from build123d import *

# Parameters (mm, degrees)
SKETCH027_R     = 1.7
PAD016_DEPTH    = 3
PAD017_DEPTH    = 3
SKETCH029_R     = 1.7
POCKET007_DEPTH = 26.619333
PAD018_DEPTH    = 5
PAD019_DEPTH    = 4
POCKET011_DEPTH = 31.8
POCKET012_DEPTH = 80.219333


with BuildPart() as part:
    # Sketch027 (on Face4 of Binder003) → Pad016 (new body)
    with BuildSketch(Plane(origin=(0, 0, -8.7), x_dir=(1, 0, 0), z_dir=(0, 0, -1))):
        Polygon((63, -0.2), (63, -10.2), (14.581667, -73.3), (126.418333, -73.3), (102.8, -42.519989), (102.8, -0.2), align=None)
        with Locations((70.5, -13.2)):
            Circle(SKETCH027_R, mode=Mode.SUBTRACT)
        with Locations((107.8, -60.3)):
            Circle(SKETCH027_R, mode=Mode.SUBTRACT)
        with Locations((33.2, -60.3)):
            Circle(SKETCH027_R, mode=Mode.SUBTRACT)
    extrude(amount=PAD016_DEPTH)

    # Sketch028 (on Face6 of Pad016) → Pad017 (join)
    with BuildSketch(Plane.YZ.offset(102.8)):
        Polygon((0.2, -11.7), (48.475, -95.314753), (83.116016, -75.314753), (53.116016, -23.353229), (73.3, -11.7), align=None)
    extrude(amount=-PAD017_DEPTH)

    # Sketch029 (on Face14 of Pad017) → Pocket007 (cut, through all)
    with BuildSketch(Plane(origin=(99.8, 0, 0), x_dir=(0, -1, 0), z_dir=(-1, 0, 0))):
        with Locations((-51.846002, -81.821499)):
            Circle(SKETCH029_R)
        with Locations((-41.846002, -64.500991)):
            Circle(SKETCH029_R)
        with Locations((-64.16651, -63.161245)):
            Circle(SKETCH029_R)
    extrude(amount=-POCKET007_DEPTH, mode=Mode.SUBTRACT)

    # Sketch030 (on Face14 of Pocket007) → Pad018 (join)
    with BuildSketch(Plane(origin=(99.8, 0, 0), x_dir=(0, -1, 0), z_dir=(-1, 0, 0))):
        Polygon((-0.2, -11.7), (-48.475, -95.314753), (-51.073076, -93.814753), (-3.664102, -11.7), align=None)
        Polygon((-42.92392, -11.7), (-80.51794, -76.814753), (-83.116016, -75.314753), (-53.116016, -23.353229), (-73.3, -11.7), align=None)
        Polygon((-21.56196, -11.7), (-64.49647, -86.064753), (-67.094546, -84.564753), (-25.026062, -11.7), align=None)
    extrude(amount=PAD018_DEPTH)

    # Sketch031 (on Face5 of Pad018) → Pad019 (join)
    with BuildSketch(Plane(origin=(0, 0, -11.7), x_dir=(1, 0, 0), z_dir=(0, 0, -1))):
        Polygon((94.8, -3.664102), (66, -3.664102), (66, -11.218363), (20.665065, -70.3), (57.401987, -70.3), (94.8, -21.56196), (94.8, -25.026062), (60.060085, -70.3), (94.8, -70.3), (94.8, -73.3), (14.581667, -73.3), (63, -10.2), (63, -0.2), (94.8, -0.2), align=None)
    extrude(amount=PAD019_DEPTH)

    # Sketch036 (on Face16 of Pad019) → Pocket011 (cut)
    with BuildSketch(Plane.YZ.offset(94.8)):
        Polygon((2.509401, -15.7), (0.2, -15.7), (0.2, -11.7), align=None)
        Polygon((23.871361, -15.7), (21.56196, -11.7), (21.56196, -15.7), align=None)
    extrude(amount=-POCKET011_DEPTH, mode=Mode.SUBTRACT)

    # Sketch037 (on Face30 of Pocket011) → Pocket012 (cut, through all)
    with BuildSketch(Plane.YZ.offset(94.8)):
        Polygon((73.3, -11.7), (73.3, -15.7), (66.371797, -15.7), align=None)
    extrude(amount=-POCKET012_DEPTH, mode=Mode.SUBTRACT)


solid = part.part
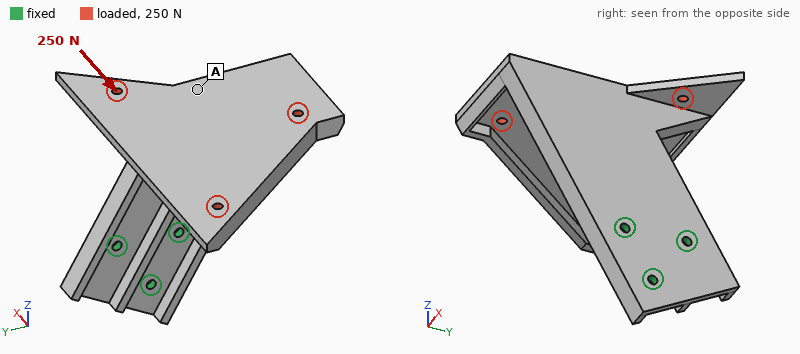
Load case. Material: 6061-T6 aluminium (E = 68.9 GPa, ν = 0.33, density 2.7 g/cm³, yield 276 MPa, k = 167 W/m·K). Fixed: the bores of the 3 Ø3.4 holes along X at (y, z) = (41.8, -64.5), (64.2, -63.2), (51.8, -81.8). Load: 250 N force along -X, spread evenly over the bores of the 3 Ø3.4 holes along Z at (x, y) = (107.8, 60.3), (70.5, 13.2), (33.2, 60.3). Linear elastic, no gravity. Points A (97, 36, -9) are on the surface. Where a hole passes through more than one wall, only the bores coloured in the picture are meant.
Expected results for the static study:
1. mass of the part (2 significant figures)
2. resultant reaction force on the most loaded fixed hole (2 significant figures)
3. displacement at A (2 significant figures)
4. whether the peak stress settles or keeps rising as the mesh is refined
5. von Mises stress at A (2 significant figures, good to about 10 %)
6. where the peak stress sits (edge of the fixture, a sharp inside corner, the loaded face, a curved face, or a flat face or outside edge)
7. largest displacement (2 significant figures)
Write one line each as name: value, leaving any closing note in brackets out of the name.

mass of the part: 85 g
resultant reaction force on the most loaded fixed hole: 400 N
displacement at A: 0.60 mm
whether the peak stress settles or keeps rising as the mesh is refined: keeps rising
von Mises stress at A: 13 MPa
where the peak stress sits: edge of the fixture
largest displacement: 1.7 mm
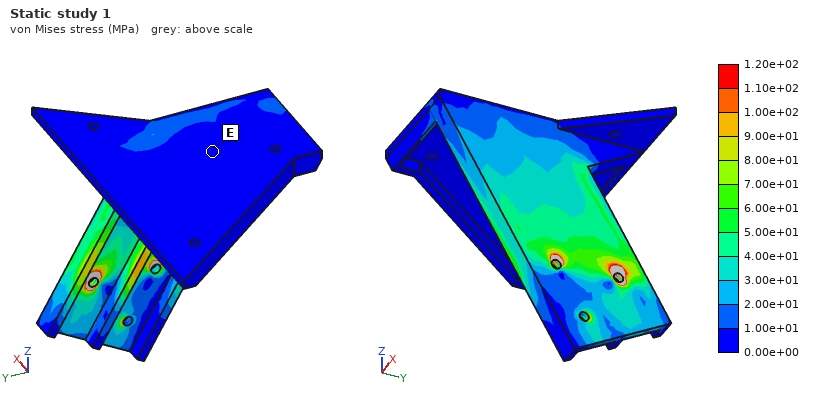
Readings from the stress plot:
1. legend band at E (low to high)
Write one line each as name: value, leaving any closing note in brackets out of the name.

legend band at E: 0.00e+00 to 1.00e+01 MPa
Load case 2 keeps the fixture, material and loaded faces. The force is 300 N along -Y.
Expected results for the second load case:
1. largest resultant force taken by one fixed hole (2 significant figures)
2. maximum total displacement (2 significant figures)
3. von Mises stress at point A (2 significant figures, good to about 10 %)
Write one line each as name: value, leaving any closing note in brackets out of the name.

largest resultant force taken by one fixed hole: 850 N
maximum total displacement: 1.6 mm
von Mises stress at point A: 30 MPa
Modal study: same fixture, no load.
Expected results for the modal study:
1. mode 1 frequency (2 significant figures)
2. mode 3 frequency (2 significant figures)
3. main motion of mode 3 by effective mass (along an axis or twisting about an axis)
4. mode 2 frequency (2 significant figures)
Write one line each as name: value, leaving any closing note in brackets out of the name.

mode 1 frequency: 300 Hz
mode 3 frequency: 810 Hz
main motion of mode 3 by effective mass: along X
mode 2 frequency: 480 Hz
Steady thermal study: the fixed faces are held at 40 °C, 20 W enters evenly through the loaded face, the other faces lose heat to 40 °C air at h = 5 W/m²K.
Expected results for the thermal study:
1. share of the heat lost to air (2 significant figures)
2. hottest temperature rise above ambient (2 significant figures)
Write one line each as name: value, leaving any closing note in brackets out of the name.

share of the heat lost to air: 16 %
hottest temperature rise above ambient: 56 K
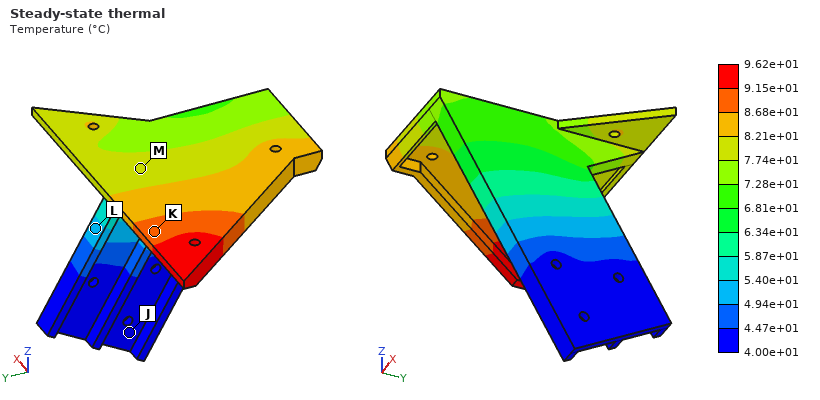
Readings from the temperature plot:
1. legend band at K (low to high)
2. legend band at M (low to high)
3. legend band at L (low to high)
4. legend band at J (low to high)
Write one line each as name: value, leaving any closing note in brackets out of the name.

legend band at K: 8.68e+01 to 9.15e+01 °C
legend band at M: 7.74e+01 to 8.21e+01 °C
legend band at L: 4.94e+01 to 5.40e+01 °C
legend band at J: 4.00e+01 to 4.47e+01 °C
